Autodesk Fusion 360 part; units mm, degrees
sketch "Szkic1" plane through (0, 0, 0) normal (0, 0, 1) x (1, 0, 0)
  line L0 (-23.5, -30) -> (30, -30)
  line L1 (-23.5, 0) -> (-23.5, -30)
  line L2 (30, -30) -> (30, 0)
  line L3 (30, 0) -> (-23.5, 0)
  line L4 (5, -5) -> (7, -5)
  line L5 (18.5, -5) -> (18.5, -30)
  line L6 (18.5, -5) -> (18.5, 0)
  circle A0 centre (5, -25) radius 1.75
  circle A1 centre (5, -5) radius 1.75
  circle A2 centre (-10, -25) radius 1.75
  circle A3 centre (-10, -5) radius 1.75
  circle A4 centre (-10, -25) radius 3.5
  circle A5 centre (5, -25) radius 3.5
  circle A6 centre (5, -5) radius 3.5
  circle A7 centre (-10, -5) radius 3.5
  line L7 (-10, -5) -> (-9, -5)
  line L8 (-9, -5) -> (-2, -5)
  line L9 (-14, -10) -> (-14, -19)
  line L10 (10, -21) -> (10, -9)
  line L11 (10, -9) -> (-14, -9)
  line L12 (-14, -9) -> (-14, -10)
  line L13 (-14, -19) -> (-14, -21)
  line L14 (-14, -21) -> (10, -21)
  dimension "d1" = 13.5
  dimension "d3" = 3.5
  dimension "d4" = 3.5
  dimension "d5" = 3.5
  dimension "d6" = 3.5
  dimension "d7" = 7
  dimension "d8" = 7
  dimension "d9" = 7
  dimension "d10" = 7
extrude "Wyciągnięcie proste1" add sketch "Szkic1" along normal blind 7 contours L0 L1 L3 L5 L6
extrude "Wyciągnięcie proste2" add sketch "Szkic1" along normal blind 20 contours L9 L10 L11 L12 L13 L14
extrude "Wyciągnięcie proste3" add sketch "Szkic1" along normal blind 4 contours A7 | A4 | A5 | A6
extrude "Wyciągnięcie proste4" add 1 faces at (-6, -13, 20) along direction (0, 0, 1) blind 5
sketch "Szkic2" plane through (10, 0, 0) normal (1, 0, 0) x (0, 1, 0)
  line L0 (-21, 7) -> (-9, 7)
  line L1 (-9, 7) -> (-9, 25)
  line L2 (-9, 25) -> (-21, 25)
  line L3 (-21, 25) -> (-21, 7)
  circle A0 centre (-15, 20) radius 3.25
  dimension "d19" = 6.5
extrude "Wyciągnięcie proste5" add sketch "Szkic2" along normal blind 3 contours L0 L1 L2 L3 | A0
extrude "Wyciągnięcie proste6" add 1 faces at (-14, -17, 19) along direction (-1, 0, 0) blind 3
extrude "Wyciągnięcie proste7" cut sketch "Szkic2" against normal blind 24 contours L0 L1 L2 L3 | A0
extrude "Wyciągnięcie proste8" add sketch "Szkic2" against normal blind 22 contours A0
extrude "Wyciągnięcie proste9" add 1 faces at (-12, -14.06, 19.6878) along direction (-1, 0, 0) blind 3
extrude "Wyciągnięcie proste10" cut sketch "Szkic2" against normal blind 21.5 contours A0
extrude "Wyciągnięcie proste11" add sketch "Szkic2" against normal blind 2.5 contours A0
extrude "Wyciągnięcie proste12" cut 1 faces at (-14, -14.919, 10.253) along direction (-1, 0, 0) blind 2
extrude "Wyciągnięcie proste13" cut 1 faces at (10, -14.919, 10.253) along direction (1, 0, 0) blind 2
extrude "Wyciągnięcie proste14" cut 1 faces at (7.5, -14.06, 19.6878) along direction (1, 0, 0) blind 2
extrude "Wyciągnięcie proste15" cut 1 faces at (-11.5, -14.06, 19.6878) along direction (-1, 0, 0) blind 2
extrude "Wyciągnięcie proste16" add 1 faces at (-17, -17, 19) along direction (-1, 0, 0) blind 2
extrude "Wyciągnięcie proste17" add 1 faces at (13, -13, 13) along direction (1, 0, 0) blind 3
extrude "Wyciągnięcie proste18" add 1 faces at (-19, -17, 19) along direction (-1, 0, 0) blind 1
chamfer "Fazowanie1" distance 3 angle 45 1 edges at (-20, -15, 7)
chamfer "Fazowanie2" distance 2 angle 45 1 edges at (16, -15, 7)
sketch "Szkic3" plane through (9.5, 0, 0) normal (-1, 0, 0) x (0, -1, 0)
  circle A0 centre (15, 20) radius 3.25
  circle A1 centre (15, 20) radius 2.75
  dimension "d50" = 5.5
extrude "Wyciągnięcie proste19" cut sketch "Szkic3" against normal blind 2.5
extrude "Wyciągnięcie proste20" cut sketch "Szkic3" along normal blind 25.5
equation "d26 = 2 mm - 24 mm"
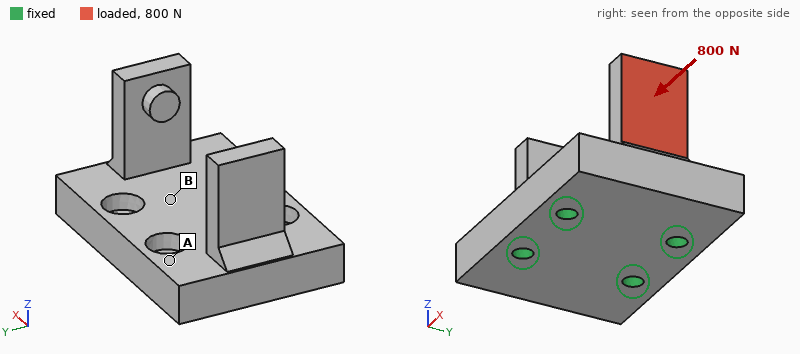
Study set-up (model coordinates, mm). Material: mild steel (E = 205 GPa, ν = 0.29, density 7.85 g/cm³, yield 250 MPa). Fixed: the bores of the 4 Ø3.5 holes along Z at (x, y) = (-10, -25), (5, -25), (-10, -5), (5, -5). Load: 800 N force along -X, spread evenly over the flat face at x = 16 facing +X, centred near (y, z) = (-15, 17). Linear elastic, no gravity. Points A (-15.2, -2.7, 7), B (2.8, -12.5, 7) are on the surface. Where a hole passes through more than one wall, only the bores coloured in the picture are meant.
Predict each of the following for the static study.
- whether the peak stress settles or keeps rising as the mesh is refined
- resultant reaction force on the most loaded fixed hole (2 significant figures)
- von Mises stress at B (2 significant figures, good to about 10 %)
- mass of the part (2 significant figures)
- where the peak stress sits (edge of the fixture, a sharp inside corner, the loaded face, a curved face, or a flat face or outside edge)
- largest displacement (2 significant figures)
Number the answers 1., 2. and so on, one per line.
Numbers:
1. keeps rising
2. 450 N
3. 36 MPa
4. 80 g
5. a sharp inside corner
6. 75 µm
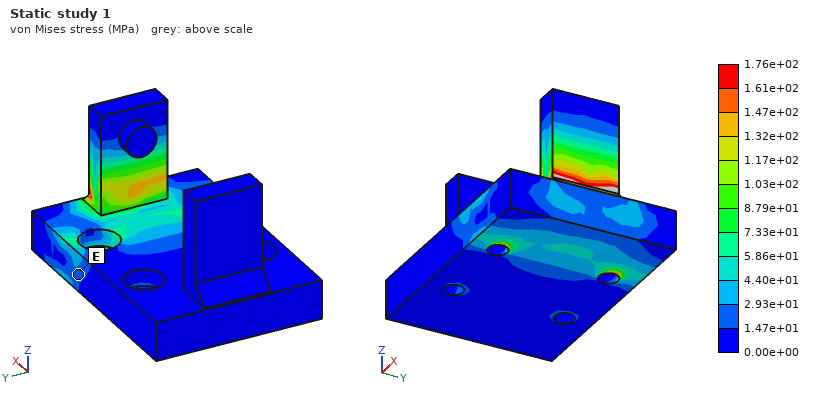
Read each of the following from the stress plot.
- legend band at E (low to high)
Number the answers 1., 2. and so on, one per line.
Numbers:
1. 1.47e+01 to 2.93e+01 MPa
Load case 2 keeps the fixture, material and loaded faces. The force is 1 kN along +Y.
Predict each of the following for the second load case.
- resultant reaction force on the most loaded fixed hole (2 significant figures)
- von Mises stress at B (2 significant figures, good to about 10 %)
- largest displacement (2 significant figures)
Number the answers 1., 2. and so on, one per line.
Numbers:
1. 1.0 kN
2. 16 MPa
3. 24 µm
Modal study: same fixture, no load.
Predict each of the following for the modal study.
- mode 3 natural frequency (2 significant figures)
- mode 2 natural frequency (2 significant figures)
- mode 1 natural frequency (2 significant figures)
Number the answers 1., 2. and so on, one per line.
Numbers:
1. 15 kHz
2. 8100 Hz
3. 7600 Hz
